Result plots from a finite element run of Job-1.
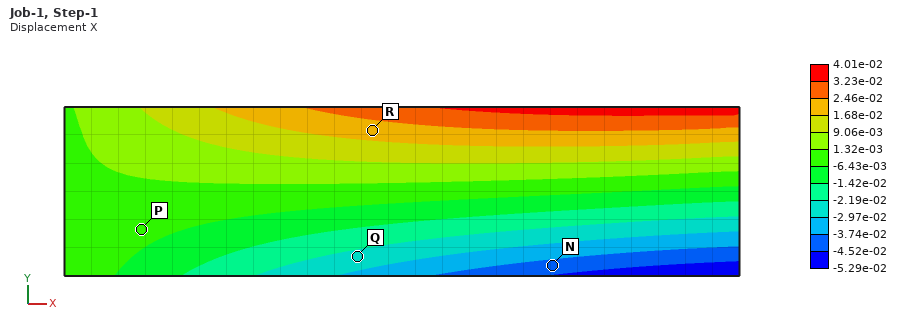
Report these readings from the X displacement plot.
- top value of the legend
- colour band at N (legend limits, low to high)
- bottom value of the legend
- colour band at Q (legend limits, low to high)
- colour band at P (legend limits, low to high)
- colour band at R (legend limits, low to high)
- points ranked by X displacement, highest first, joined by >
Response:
4.01e-02
-4.52e-02 to -3.74e-02
-5.29e-02
-2.97e-02 to -2.19e-02
-6.43e-03 to 1.32e-03
1.68e-02 to 2.46e-02
R > P > Q > N
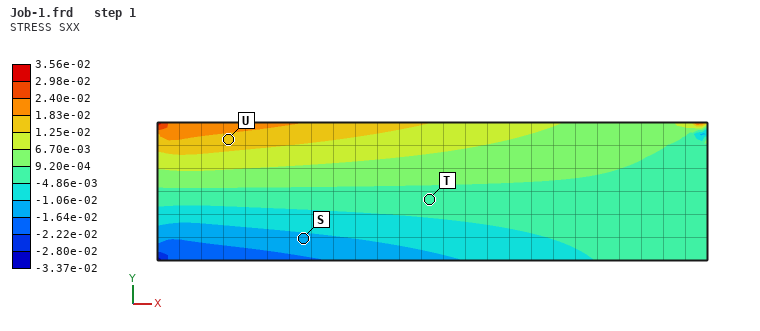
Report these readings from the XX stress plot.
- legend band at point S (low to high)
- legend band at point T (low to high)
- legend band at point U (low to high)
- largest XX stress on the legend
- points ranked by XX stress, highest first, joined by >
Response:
-1.64e-02 to -1.06e-02
-4.86e-03 to 9.20e-04
1.25e-02 to 1.83e-02
3.56e-02
U > T > S
